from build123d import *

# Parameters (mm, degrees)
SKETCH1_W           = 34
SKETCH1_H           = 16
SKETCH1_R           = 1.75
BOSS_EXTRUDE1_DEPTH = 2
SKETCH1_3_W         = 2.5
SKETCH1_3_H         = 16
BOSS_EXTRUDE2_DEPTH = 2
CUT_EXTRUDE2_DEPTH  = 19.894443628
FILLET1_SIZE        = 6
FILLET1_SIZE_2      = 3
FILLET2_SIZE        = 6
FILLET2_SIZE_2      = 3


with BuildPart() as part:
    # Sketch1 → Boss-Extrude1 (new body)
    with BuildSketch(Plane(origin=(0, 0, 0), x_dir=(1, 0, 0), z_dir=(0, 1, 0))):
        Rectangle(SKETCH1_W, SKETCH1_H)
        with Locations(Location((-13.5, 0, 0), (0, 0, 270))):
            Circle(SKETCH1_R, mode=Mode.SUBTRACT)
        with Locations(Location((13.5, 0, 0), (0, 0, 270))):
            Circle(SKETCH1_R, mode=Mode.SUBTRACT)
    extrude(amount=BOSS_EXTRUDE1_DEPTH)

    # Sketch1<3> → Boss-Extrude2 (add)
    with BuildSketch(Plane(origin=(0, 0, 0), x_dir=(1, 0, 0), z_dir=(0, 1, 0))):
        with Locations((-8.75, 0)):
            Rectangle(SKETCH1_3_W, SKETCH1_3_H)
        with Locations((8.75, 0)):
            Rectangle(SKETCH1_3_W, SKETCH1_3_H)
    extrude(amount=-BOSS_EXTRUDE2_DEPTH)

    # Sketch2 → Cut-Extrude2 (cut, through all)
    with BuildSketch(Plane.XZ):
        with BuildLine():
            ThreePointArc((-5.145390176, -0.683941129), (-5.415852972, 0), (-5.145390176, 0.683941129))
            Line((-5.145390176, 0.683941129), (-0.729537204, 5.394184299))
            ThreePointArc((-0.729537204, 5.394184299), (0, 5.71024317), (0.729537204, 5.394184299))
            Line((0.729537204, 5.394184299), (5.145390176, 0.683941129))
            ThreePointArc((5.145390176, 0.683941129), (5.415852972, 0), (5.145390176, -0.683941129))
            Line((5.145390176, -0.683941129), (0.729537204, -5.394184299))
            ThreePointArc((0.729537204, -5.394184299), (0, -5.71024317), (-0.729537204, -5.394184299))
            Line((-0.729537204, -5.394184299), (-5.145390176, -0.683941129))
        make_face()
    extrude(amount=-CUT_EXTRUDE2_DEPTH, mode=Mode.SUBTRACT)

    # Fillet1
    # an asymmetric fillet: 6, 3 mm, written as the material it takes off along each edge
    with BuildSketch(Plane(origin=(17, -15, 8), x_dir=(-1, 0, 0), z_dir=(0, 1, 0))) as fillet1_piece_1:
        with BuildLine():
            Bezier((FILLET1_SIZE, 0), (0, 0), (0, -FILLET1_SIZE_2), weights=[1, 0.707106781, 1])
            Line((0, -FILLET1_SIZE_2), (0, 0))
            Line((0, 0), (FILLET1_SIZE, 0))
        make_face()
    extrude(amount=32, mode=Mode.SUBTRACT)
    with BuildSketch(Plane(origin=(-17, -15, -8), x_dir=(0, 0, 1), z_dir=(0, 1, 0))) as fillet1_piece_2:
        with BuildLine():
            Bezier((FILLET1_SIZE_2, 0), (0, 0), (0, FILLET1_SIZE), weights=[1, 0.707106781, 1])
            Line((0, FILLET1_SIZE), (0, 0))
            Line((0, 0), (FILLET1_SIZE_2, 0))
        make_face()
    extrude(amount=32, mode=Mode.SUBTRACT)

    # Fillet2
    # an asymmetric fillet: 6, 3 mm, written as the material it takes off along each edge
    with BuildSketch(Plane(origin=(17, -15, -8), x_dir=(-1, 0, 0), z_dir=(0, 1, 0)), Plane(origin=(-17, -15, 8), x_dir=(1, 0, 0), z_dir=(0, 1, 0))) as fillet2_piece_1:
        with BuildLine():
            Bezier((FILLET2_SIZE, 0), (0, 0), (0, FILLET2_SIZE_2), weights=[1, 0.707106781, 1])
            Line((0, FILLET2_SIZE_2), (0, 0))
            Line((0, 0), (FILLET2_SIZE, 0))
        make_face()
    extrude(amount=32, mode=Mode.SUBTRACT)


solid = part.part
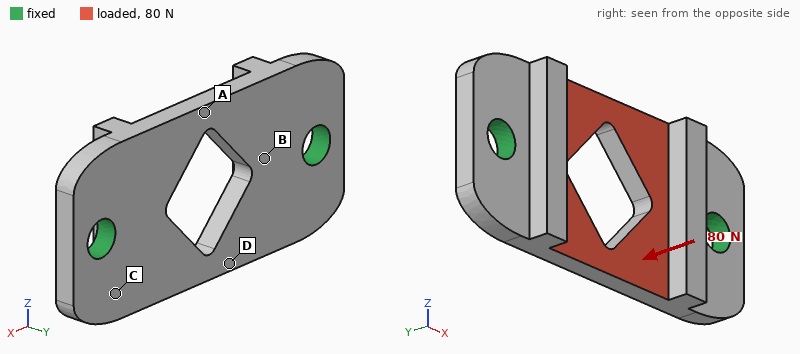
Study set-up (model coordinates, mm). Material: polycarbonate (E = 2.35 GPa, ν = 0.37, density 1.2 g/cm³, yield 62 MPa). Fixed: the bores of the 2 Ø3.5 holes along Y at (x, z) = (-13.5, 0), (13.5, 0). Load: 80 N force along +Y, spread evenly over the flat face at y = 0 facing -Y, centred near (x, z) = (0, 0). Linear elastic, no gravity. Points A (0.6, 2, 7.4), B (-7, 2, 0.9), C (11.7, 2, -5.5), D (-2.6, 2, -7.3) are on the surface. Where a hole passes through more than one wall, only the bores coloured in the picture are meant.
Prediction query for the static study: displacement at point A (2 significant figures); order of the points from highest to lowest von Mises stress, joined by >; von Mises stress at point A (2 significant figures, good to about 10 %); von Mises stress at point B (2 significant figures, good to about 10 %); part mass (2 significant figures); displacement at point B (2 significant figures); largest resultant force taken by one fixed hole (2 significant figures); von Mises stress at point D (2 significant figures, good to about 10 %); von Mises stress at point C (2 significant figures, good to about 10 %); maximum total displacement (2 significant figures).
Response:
0.32 mm
A > D > C > B
21 MPa
4.4 MPa
1.2 g
0.14 mm
40 N
14 MPa
10 MPa
0.33 mm
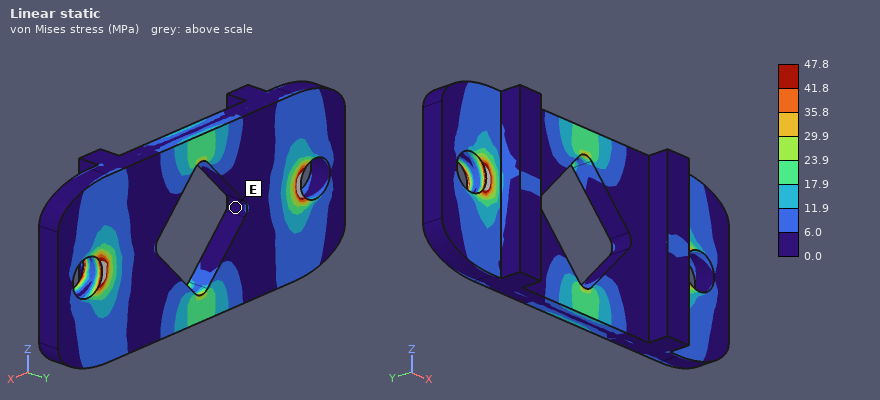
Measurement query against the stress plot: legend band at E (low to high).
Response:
0.0 to 6.0 MPa
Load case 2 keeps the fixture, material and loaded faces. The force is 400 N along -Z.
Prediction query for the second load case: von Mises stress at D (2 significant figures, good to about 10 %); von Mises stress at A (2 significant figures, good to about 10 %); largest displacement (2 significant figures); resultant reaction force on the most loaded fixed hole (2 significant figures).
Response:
24 MPa
24 MPa
0.30 mm
200 N
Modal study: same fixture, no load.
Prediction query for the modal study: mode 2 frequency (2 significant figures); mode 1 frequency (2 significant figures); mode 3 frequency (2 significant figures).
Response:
4300 Hz
4200 Hz
7300 Hz
